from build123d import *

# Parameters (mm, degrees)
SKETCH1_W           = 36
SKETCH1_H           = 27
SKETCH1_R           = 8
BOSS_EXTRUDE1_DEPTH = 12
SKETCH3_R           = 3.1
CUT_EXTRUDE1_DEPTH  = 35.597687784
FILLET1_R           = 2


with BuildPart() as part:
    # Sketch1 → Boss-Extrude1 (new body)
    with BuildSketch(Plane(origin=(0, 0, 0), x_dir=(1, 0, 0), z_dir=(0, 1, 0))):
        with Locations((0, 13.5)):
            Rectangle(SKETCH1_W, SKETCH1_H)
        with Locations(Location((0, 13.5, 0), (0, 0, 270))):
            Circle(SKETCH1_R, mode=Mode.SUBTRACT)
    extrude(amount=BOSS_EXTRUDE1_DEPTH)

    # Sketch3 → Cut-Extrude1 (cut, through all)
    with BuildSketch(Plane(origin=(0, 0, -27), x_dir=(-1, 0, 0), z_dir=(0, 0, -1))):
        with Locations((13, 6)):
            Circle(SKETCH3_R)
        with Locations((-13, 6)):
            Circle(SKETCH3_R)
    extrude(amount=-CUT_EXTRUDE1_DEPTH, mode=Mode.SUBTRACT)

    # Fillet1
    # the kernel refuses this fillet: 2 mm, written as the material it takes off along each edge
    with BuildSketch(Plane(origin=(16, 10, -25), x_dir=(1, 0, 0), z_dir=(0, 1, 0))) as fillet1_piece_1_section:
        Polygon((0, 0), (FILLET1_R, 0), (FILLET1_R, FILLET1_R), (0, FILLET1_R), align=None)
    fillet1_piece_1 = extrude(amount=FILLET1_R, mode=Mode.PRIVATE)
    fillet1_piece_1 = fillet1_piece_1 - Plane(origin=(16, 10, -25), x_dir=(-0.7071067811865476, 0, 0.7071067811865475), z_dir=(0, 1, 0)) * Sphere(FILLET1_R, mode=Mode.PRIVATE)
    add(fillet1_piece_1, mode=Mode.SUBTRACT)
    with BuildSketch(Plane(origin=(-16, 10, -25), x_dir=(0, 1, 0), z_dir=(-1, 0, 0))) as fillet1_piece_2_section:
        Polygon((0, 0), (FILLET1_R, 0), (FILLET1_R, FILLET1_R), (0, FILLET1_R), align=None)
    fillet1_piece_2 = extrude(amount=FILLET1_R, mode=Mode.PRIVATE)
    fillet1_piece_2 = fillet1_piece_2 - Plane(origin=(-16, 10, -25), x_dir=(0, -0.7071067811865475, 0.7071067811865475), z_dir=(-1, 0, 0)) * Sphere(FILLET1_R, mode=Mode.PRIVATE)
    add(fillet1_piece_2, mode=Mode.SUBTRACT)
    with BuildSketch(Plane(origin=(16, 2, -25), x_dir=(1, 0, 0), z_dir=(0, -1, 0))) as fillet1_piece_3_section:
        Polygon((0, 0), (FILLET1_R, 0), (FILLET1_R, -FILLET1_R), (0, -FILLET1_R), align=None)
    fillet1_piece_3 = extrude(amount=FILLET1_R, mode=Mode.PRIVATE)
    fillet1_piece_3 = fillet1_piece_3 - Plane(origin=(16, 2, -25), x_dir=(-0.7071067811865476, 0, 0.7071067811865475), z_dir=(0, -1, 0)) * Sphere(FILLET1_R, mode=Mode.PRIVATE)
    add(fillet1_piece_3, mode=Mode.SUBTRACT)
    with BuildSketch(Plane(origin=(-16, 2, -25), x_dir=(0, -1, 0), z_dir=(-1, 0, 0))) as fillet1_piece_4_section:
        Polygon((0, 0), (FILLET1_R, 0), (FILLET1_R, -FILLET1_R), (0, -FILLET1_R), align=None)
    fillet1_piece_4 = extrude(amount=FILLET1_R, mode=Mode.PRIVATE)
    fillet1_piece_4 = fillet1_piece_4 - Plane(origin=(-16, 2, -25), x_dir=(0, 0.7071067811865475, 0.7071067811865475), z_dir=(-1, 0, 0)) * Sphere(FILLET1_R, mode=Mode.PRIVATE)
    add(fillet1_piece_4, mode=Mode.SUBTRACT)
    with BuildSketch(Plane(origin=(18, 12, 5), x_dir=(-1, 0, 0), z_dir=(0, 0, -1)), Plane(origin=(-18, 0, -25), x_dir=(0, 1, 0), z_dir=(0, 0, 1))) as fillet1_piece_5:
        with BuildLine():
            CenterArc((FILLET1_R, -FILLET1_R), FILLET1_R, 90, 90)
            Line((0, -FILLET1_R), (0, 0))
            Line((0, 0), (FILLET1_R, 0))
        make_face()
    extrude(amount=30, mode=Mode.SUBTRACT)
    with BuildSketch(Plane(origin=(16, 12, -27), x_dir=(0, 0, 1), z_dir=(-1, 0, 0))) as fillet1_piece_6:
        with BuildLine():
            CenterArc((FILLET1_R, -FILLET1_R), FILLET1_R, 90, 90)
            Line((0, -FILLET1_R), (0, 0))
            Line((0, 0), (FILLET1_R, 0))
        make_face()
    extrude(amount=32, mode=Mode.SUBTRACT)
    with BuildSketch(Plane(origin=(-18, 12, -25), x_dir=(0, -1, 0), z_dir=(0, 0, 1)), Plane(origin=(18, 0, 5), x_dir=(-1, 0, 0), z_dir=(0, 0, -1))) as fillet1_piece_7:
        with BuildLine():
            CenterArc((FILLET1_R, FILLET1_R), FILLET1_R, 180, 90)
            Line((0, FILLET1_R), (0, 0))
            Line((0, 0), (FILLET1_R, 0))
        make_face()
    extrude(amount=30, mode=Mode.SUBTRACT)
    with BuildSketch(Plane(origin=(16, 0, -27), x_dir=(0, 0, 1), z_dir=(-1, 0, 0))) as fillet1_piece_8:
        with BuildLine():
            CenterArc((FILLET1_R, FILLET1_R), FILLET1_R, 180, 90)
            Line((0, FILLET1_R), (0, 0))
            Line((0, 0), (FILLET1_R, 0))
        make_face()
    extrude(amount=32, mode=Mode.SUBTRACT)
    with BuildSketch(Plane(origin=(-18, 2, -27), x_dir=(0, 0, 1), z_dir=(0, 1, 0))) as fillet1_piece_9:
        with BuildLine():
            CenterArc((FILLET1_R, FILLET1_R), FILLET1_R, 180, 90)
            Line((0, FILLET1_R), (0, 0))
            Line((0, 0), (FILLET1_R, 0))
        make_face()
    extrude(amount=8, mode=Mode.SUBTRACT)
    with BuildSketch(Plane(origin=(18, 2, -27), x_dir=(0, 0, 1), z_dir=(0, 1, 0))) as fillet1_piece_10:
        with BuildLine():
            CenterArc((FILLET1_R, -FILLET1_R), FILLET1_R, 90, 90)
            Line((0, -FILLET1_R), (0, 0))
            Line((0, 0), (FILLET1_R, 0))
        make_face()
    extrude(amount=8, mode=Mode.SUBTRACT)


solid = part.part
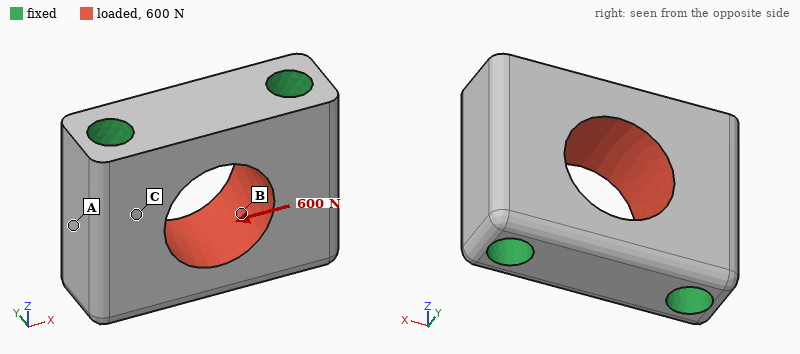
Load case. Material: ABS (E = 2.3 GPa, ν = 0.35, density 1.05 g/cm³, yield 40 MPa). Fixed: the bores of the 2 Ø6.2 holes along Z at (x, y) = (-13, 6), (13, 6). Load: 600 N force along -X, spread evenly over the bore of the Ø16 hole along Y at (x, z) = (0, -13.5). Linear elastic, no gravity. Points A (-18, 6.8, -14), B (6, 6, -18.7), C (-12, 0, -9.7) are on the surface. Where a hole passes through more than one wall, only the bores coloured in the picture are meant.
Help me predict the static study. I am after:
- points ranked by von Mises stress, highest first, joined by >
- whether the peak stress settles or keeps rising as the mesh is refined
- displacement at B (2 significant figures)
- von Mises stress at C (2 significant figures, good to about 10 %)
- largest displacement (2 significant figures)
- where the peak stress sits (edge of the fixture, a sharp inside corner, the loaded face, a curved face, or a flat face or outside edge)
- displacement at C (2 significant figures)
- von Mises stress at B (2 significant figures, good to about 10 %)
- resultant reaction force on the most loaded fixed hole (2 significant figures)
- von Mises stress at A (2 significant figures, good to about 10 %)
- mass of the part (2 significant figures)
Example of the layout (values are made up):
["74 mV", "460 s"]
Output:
["B > C > A", "keeps rising", "2.3 µm", "0.64 MPa", "4.9 µm", "edge of the fixture", "1.5 µm", "1.7 MPa", "300 N", "0.25 MPa", "7.8 g"]
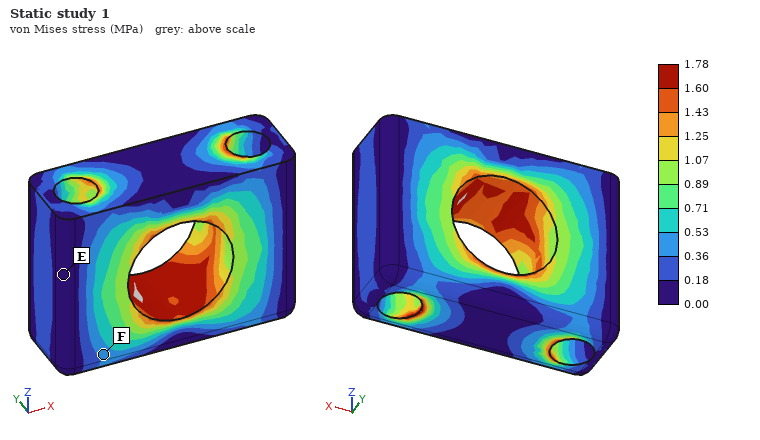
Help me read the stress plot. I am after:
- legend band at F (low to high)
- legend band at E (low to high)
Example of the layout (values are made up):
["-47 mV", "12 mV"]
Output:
["0.36 to 0.53 MPa", "0.00 to 0.18 MPa"]
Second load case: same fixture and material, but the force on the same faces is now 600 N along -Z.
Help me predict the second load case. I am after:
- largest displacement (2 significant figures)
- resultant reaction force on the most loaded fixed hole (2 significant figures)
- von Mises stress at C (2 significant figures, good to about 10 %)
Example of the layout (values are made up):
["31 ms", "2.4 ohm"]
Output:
["15 µm", "300 N", "0.79 MPa"]
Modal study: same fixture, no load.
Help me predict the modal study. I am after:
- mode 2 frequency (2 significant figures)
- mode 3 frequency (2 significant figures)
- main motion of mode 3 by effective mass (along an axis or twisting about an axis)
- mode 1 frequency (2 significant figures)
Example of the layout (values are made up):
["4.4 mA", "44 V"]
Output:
["18 kHz", "20 kHz", "along Z", "17 kHz"]
